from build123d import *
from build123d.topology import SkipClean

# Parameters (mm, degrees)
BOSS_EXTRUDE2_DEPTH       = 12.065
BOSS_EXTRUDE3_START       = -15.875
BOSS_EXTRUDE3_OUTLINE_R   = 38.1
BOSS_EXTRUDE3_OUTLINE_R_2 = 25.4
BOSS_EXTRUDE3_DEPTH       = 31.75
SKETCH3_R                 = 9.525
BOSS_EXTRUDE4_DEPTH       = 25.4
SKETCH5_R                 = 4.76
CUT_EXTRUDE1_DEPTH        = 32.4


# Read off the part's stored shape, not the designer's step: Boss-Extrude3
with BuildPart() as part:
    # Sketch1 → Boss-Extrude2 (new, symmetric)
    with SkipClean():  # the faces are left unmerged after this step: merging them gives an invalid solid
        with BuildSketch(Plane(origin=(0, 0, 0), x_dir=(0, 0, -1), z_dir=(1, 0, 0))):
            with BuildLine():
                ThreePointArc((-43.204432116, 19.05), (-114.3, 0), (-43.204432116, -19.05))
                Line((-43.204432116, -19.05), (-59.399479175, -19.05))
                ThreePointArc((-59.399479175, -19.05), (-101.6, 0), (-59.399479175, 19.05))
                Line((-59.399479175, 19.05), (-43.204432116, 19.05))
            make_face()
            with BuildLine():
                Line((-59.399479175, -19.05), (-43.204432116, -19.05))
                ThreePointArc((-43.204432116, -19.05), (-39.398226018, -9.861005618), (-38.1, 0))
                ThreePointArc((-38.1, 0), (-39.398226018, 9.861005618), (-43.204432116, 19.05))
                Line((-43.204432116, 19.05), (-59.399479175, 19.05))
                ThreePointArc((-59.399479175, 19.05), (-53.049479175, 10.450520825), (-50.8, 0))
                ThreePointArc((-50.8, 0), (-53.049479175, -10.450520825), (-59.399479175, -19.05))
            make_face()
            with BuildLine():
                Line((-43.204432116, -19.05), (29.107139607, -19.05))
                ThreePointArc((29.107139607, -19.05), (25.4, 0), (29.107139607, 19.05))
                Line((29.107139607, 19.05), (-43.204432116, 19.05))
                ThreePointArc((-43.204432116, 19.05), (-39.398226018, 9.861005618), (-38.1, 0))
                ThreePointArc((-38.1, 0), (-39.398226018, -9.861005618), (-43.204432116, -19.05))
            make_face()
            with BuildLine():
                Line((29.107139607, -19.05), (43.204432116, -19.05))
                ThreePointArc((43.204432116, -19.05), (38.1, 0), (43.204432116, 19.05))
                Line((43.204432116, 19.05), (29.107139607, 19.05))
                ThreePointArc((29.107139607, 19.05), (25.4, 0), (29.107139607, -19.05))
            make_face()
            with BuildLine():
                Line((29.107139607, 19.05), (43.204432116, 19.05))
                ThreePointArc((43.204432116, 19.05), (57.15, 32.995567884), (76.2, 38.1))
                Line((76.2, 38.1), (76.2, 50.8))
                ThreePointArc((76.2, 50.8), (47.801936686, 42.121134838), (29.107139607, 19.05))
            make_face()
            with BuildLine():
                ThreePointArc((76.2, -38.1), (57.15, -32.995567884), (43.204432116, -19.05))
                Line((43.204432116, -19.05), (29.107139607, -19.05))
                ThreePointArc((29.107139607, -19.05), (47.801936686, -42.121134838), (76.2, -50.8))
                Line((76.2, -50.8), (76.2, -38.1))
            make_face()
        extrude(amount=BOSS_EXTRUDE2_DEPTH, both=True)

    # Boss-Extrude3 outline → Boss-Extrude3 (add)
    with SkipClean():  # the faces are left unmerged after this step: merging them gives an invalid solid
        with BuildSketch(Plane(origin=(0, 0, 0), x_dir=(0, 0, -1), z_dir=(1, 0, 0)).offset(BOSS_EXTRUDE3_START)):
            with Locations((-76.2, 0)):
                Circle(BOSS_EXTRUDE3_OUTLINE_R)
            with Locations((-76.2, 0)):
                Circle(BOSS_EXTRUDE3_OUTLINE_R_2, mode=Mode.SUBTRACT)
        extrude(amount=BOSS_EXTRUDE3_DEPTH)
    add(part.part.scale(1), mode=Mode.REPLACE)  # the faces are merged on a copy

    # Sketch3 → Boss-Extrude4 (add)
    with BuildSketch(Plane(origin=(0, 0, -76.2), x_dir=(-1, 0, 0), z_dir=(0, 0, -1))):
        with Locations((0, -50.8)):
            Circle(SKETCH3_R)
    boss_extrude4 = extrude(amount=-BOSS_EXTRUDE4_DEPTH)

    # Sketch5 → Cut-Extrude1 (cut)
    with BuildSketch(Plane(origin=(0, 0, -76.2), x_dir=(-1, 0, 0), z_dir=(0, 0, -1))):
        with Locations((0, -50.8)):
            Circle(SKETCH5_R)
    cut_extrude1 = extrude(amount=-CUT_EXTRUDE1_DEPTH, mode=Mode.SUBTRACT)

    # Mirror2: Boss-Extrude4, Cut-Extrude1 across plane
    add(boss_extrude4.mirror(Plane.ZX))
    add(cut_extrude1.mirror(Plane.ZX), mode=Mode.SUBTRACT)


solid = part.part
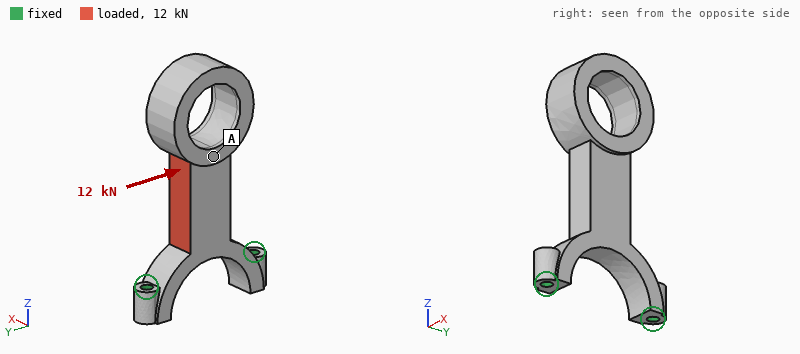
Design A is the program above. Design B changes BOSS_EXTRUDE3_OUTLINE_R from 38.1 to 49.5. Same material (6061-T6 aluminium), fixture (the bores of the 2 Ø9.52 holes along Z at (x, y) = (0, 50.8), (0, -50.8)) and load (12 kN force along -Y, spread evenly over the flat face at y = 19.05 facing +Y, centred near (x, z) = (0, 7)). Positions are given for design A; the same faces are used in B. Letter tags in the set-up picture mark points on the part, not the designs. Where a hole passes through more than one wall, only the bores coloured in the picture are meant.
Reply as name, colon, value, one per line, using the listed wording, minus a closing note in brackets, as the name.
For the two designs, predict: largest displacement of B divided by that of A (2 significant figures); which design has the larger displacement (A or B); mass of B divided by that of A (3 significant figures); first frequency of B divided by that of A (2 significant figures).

largest displacement of B divided by that of A: 0.82
which design has the larger displacement: A
mass of B divided by that of A: 1.47
first frequency of B divided by that of A: 0.70
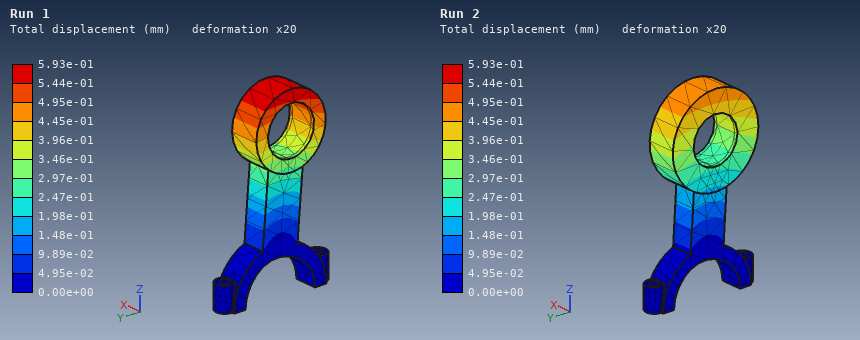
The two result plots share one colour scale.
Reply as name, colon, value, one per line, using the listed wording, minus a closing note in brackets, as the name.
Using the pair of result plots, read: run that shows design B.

run that shows design B: Run 2
